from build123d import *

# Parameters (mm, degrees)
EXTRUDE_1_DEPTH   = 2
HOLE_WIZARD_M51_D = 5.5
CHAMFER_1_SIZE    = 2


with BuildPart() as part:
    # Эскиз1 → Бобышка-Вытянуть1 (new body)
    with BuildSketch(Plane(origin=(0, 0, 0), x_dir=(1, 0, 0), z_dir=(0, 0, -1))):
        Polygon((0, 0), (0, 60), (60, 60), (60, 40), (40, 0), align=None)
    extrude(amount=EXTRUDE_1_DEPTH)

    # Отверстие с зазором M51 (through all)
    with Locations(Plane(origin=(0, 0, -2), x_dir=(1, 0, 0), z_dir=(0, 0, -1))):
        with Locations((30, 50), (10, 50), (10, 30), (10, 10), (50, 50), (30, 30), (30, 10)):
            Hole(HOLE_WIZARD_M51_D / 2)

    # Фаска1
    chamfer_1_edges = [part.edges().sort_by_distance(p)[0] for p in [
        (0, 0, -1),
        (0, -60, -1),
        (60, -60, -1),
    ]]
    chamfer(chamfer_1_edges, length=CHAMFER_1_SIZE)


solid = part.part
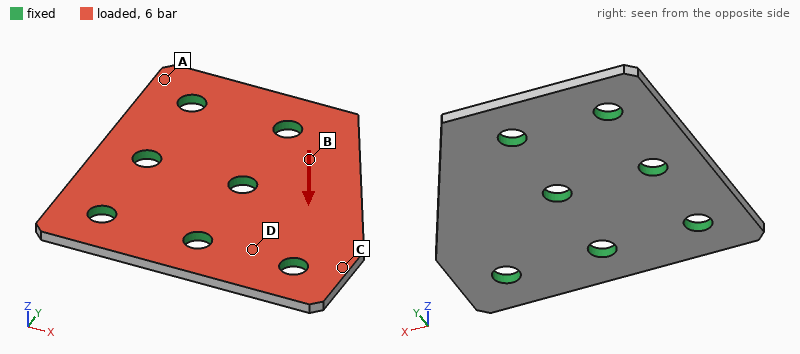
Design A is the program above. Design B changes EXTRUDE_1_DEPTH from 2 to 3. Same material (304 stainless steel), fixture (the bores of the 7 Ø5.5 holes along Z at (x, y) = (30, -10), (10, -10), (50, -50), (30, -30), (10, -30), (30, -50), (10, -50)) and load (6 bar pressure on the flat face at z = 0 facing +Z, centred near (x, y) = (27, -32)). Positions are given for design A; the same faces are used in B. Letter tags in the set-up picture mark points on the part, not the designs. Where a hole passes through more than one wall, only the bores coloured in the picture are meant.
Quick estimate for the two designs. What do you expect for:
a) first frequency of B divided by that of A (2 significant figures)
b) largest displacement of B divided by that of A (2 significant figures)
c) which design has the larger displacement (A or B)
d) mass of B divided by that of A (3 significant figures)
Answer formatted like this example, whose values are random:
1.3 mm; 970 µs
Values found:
1.4; 0.31; A; 1.50
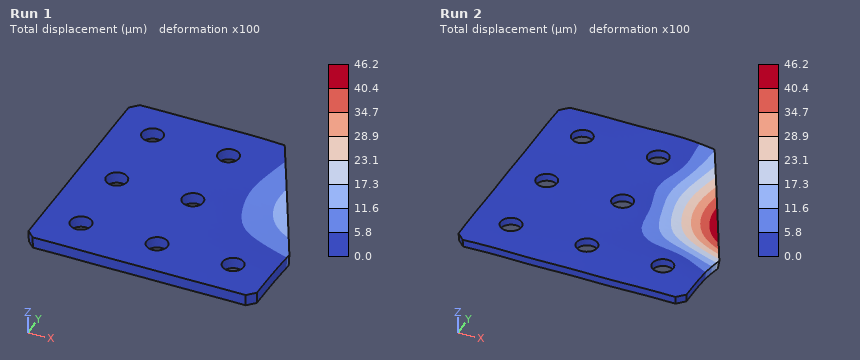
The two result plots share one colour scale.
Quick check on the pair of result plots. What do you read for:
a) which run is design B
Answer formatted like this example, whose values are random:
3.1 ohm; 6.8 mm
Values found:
Run 1
